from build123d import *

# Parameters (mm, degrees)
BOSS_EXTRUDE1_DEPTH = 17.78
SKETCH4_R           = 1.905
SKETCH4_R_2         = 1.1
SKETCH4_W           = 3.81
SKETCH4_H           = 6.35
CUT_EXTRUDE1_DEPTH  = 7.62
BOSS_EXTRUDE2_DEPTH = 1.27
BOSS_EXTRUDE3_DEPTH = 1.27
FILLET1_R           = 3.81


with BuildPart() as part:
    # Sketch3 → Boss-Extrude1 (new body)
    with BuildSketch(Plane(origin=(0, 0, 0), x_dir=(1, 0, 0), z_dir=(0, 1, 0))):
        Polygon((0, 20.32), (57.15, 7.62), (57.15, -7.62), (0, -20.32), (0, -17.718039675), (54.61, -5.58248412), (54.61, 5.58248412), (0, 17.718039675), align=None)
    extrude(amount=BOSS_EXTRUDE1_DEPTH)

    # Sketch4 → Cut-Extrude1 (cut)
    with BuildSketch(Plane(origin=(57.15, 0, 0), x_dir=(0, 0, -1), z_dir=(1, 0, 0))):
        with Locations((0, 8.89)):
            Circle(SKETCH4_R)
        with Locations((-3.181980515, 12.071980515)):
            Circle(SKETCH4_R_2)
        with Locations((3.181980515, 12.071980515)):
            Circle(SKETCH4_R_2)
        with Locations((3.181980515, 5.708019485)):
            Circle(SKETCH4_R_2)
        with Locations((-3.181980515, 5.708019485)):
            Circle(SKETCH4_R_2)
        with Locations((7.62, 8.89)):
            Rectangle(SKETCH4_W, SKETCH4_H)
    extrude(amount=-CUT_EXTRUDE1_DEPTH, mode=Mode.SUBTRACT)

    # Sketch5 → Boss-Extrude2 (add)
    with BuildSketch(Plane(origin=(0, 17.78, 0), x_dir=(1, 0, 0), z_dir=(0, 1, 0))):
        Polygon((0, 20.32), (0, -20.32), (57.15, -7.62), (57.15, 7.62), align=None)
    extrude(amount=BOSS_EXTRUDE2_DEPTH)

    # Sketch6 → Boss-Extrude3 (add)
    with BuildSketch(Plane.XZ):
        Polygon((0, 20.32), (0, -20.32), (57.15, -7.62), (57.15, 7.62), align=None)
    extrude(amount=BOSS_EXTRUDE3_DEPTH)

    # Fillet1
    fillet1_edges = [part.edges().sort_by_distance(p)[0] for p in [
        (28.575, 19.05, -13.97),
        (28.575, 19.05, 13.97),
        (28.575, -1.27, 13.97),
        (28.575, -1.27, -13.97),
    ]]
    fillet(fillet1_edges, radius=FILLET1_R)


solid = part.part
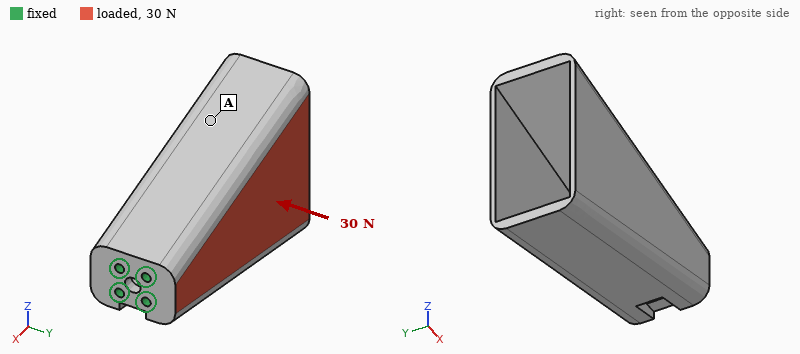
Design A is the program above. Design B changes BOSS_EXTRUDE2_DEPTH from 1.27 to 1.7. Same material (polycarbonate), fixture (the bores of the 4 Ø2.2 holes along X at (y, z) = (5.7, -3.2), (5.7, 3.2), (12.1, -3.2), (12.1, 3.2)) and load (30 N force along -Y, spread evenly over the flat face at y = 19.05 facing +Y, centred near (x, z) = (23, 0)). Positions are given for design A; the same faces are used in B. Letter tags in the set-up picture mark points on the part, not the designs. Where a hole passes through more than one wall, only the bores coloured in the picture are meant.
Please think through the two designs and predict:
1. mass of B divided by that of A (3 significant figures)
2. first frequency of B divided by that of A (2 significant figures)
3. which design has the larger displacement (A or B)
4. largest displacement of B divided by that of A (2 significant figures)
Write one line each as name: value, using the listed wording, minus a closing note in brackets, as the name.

mass of B divided by that of A: 1.08
first frequency of B divided by that of A: 0.97
which design has the larger displacement: A
largest displacement of B divided by that of A: 0.77
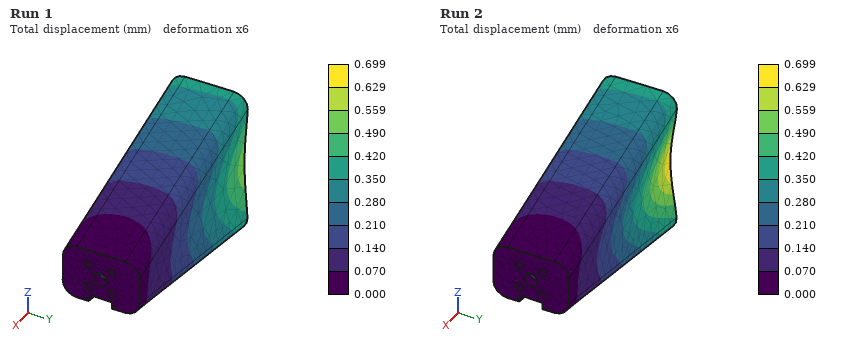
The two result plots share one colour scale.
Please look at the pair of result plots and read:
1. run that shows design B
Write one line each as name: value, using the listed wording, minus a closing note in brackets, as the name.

run that shows design B: Run 1
